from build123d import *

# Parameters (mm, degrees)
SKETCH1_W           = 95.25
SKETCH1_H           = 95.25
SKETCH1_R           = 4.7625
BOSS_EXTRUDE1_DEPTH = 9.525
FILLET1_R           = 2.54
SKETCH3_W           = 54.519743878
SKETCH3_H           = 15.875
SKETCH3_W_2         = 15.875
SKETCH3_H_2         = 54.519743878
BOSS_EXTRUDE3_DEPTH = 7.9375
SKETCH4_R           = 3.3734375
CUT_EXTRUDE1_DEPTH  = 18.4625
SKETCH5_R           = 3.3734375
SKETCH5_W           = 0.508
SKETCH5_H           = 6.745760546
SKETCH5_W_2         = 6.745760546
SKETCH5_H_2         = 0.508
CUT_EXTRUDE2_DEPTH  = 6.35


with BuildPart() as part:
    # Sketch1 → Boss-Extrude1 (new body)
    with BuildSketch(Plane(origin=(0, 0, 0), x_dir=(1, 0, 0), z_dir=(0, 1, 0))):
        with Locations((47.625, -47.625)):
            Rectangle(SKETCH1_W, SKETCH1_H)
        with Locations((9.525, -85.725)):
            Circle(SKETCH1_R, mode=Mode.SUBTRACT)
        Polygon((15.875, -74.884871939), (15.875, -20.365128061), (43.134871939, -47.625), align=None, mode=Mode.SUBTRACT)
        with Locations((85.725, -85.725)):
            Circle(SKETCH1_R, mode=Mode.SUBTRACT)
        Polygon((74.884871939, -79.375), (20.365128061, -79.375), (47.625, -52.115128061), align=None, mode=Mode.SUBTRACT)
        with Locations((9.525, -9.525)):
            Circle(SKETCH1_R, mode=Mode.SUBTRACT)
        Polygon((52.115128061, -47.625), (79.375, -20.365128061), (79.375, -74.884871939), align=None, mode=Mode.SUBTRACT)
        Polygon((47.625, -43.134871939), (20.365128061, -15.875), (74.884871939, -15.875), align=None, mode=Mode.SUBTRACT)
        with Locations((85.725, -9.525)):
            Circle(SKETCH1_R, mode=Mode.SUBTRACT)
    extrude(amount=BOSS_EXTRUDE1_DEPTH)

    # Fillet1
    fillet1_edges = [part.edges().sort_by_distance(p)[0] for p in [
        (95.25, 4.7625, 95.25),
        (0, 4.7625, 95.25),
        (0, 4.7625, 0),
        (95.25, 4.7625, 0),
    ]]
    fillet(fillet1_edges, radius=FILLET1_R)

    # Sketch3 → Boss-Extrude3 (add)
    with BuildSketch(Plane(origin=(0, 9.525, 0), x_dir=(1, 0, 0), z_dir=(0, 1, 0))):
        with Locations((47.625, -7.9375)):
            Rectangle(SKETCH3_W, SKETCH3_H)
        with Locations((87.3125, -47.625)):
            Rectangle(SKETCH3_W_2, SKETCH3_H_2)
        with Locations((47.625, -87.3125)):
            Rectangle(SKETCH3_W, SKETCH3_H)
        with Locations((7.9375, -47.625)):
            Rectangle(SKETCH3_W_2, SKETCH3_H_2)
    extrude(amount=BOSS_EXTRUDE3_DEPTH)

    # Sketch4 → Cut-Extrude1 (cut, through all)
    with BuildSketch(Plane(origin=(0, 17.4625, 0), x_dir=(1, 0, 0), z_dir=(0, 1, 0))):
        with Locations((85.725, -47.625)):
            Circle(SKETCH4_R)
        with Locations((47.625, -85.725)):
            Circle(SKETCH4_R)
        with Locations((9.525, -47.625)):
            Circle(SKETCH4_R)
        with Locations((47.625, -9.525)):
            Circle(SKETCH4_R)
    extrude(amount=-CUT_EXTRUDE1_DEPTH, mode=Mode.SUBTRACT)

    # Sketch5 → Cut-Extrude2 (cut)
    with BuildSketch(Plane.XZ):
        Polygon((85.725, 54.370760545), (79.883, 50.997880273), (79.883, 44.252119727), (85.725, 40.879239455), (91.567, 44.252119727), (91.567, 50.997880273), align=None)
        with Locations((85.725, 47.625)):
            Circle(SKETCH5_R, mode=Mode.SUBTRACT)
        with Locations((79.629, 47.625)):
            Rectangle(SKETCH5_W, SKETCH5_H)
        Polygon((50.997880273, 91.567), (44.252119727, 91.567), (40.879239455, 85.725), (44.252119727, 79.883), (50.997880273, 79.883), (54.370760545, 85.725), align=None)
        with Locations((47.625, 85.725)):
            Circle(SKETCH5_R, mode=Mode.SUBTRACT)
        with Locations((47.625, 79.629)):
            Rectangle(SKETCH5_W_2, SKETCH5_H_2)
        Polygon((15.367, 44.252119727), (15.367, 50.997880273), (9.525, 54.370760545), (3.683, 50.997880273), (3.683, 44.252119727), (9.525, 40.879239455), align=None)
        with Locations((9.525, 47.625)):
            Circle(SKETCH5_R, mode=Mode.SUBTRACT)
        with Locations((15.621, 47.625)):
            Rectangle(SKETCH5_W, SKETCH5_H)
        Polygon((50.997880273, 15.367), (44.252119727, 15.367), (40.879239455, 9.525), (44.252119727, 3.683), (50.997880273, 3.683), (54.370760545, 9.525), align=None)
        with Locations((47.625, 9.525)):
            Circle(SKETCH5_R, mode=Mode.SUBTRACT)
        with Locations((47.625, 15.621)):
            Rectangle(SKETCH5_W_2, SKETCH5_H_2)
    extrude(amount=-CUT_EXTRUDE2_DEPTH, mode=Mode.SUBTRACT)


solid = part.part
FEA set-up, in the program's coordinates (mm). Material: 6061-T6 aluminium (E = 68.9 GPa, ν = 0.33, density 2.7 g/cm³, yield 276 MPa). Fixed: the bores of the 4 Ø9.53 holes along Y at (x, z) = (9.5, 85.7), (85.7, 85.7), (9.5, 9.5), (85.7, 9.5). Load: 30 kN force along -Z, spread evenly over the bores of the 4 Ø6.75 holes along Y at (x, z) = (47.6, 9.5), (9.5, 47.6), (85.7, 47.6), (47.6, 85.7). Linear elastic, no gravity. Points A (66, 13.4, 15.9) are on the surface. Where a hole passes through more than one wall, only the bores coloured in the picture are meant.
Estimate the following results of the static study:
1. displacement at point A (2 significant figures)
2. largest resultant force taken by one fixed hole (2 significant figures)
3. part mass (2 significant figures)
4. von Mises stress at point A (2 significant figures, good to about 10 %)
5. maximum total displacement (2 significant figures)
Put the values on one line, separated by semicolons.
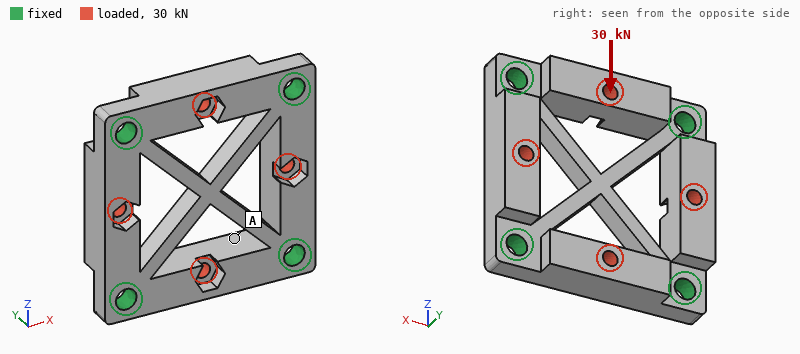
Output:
0.062 mm; 7.7 kN; 210 g; 23 MPa; 0.11 mm
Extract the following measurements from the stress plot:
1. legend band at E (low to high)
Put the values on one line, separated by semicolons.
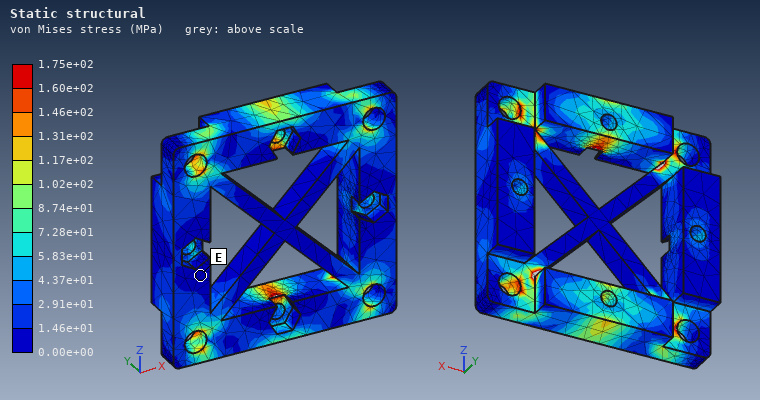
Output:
0.00e+00 to 1.46e+01 MPa
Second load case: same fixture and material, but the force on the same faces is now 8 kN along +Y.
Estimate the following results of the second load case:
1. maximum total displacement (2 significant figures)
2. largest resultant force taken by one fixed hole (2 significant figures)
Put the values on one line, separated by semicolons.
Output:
27 µm; 2.8 kN
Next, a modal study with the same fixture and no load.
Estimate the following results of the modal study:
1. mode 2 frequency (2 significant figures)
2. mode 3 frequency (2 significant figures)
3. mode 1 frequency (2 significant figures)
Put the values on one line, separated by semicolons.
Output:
9400 Hz; 10 kHz; 5700 Hz
